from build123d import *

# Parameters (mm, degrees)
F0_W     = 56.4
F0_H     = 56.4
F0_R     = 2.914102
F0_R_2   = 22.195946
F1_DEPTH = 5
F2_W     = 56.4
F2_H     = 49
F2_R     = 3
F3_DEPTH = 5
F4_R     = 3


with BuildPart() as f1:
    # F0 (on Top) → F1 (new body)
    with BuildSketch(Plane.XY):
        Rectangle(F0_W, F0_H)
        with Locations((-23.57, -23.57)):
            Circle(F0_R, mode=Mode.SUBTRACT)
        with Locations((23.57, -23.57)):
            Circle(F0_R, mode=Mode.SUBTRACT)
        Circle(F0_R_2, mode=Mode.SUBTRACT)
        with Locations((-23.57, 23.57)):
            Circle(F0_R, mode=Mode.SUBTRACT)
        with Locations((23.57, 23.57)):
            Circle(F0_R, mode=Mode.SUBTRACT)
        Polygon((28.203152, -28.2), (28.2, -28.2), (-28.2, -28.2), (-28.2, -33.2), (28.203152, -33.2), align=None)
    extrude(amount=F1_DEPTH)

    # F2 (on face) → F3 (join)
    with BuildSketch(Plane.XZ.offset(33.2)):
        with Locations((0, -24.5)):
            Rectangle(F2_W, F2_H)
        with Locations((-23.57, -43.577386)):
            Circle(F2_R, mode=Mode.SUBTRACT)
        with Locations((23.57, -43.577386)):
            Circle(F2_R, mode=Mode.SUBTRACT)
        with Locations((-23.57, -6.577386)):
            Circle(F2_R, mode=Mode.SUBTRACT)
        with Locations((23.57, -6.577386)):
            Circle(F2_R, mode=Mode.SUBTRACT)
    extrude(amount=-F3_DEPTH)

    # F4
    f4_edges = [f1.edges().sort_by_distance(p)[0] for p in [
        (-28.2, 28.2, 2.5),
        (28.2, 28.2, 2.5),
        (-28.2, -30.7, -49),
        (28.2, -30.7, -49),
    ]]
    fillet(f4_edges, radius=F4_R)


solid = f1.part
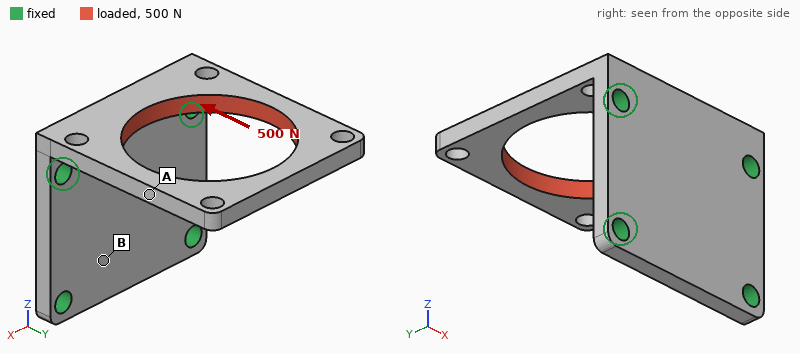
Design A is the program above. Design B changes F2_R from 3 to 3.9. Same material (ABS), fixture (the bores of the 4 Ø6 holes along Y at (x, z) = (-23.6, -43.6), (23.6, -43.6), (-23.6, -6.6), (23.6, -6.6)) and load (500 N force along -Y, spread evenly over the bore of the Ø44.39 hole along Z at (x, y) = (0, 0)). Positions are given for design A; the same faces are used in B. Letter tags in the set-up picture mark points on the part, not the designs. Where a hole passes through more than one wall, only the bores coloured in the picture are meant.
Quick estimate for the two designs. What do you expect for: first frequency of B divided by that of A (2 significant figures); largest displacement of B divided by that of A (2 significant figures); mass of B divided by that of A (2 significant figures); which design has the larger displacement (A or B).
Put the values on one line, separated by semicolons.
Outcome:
1.0; 0.80; 0.98; A
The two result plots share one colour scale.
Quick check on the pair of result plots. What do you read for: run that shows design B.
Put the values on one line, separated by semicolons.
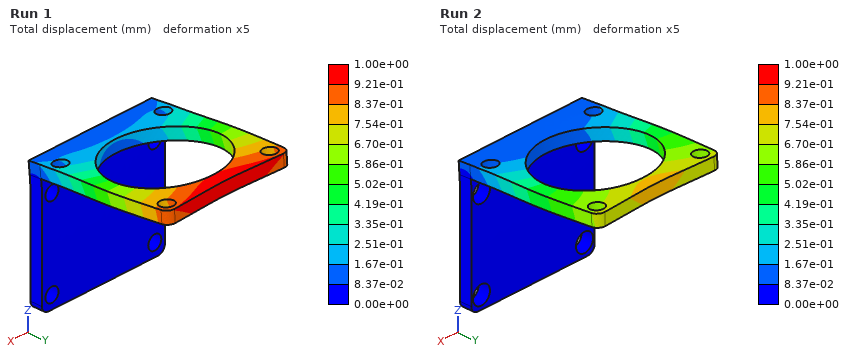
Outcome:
Run 2
